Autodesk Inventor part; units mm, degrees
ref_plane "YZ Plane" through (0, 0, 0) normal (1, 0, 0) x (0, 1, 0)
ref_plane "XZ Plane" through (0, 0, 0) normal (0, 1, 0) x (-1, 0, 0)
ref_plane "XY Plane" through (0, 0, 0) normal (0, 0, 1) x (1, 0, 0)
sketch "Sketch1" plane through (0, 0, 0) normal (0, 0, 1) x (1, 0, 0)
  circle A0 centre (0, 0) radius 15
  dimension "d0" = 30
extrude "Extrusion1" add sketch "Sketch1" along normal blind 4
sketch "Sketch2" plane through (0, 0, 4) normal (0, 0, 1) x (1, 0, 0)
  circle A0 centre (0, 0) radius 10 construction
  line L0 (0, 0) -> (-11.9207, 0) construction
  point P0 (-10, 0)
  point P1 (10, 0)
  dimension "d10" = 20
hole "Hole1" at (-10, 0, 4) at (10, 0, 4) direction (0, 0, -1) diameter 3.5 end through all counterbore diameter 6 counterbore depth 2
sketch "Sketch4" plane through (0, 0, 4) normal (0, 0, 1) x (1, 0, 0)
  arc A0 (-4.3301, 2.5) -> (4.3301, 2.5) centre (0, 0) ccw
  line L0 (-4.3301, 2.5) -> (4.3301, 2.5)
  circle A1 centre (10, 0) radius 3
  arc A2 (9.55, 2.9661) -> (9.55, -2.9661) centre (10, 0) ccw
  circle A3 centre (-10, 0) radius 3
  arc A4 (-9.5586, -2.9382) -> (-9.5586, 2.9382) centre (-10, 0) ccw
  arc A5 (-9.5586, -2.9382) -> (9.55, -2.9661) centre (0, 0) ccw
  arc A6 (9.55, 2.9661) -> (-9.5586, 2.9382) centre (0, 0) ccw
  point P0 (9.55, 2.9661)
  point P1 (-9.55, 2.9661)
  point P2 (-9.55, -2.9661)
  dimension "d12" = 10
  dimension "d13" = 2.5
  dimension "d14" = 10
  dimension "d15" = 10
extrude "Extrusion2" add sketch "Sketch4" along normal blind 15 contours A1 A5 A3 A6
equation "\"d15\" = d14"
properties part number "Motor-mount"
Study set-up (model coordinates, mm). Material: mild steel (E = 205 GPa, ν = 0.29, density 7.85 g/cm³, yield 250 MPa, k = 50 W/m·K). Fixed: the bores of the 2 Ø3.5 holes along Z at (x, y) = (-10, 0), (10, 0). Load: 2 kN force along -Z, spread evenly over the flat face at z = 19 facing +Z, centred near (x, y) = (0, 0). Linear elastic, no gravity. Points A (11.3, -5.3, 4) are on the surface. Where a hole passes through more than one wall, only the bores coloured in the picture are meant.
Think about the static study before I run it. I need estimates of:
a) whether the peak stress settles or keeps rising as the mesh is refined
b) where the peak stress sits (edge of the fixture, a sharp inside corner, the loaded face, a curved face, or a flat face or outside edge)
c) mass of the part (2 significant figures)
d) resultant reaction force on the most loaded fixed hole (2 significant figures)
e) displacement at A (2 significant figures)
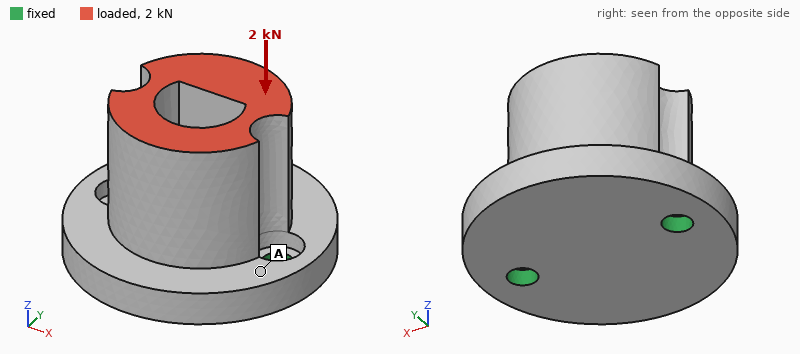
keeps rising
edge of the fixture
47 g
1.1 kN
1.1 µm
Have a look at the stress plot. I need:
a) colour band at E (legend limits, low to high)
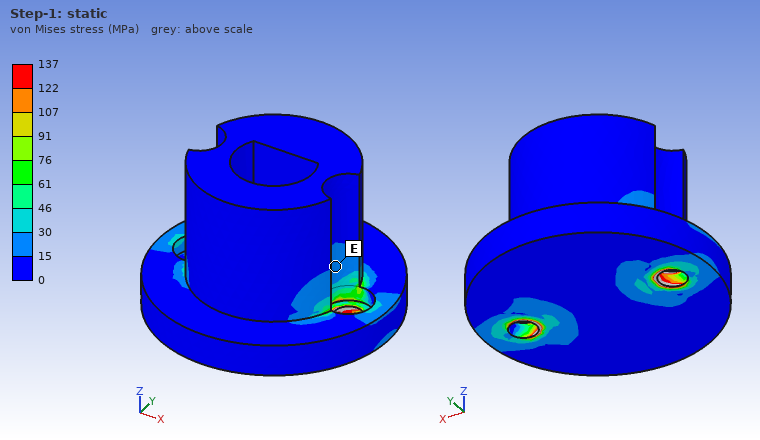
15 to 30 MPa
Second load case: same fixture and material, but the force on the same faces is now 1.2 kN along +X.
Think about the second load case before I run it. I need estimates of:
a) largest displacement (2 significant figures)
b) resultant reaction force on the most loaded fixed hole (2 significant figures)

9.2 µm
1.3 kN
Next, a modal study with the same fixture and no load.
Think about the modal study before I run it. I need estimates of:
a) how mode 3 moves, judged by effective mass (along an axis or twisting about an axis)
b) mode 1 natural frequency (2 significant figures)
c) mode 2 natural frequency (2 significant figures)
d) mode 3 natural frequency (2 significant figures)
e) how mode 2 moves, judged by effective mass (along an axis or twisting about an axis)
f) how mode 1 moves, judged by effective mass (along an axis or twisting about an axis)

along Z
5000 Hz
17 kHz
20 kHz
along X
along Y
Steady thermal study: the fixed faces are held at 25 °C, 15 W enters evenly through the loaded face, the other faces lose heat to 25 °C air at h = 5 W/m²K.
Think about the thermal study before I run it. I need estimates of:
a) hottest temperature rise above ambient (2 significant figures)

38 K
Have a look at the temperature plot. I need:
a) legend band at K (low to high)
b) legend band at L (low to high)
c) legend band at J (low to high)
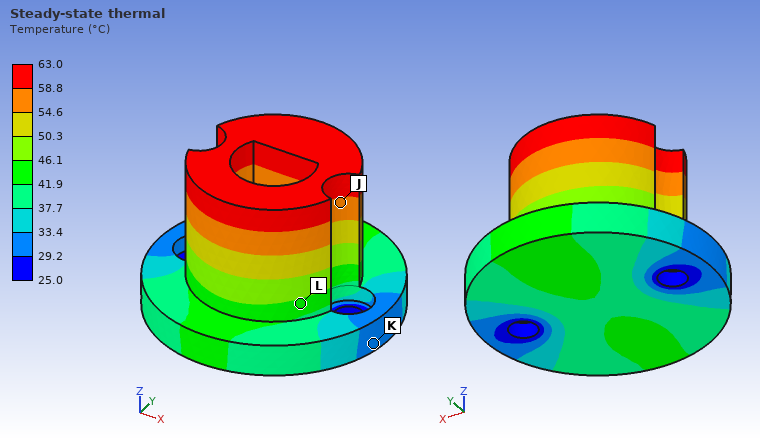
29.2 to 33.4 °C
41.9 to 46.1 °C
54.6 to 58.8 °C
